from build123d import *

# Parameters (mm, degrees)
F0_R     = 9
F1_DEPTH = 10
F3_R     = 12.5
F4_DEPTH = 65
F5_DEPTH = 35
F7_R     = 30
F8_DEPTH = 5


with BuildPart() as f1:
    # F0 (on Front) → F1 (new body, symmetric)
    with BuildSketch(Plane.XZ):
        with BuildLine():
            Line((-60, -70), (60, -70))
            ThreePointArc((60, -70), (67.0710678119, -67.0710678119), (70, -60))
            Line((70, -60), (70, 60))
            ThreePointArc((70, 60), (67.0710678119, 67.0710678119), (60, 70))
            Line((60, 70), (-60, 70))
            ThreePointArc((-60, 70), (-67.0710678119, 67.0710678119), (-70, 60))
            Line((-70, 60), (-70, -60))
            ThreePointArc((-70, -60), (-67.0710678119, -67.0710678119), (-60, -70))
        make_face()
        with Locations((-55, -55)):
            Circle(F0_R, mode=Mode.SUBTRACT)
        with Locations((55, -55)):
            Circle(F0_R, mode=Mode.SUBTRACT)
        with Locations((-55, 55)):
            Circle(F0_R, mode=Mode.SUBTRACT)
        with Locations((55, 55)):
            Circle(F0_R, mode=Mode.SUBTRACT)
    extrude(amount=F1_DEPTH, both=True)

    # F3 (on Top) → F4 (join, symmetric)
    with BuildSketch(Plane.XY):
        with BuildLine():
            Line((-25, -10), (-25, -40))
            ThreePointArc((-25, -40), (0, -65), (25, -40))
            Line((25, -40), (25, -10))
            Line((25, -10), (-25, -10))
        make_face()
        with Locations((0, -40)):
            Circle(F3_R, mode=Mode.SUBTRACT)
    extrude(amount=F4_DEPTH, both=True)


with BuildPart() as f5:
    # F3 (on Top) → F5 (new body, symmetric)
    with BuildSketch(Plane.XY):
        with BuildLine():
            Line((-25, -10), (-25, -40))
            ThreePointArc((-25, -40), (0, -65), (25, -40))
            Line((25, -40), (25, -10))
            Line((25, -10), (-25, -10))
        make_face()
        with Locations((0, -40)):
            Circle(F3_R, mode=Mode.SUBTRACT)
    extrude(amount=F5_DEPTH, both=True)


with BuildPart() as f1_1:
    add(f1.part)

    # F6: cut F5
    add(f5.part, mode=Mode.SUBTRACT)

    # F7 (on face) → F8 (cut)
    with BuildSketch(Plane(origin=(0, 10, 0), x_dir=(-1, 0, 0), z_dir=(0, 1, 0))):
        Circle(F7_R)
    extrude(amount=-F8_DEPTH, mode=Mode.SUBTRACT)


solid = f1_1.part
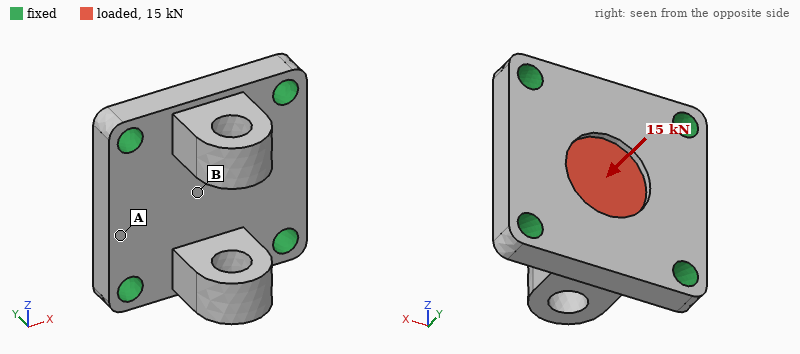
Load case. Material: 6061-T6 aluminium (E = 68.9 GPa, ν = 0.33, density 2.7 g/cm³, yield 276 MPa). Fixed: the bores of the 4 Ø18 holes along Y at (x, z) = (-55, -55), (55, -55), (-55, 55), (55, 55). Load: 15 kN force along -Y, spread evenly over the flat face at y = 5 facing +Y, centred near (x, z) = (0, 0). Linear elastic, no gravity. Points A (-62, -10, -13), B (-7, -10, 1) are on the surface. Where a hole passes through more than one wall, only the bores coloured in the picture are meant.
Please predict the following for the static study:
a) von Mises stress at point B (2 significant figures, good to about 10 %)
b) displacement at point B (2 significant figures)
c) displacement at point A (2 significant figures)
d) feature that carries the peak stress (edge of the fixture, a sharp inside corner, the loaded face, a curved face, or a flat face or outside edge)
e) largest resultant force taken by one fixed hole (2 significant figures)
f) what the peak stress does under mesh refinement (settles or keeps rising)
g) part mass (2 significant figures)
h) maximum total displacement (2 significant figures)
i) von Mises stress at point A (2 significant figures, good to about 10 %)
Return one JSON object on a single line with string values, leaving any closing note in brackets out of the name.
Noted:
{"von Mises stress at point B": "33 MPa", "displacement at point B": "49 µm", "displacement at point A": "9.6 µm", "feature that carries the peak stress": "edge of the fixture", "largest resultant force taken by one fixed hole": "4.0 kN", "what the peak stress does under mesh refinement": "keeps rising", "part mass": "1.3 kg", "maximum total displacement": "52 µm", "von Mises stress at point A": "7.6 MPa"}
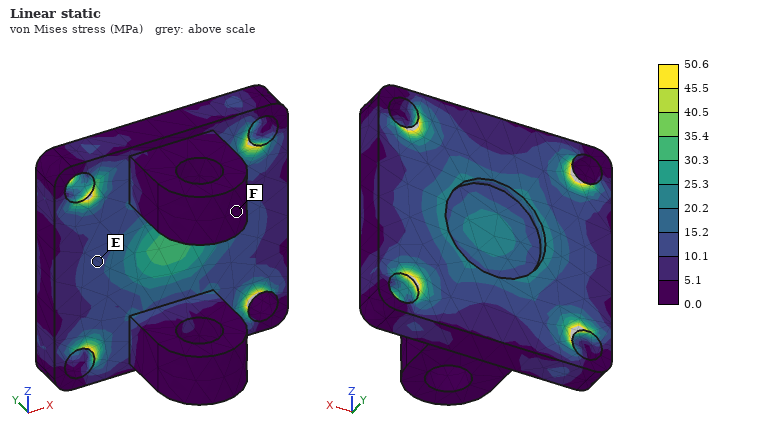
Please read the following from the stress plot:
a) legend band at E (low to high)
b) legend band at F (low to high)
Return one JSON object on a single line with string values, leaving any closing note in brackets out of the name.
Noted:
{"legend band at E": "10.1 to 15.2 MPa", "legend band at F": "0.0 to 5.1 MPa"}
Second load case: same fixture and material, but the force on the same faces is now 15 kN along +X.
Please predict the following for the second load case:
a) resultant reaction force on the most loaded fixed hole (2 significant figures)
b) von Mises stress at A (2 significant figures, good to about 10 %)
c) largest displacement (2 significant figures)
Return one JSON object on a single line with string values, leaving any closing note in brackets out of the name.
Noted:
{"resultant reaction force on the most loaded fixed hole": "4.2 kN", "von Mises stress at A": "3.1 MPa", "largest displacement": "8.9 µm"}
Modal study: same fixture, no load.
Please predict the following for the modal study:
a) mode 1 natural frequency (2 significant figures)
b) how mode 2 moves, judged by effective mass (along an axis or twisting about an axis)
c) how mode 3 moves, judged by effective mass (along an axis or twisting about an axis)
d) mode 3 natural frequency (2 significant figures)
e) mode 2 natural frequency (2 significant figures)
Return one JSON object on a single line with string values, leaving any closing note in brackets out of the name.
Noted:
{"mode 1 natural frequency": "3800 Hz", "how mode 2 moves, judged by effective mass": "along Z", "how mode 3 moves, judged by effective mass": "along Y", "mode 3 natural frequency": "6000 Hz", "mode 2 natural frequency": "4400 Hz"}
